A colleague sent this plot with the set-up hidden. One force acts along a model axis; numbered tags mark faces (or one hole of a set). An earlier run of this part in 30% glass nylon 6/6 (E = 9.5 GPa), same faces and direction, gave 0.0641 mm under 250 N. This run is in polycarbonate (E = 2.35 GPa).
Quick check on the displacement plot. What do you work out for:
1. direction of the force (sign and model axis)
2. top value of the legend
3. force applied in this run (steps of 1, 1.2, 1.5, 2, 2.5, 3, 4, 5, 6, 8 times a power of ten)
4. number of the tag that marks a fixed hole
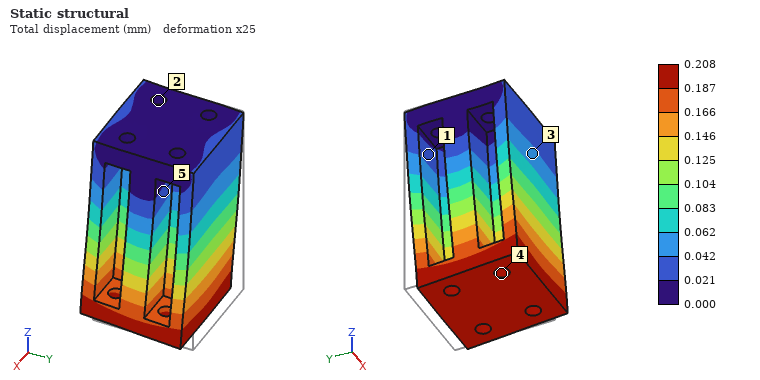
-Y
0.208 mm
200 N
2
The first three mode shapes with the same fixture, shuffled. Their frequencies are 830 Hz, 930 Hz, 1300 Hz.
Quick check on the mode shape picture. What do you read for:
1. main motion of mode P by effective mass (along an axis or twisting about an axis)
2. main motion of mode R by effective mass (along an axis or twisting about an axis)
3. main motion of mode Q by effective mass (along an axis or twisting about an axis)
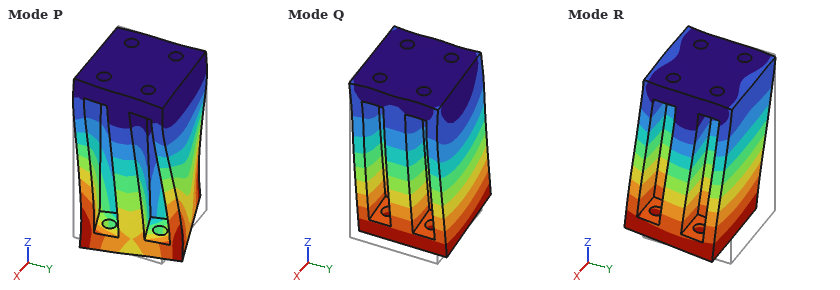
twisting about Z
along Y
along X
